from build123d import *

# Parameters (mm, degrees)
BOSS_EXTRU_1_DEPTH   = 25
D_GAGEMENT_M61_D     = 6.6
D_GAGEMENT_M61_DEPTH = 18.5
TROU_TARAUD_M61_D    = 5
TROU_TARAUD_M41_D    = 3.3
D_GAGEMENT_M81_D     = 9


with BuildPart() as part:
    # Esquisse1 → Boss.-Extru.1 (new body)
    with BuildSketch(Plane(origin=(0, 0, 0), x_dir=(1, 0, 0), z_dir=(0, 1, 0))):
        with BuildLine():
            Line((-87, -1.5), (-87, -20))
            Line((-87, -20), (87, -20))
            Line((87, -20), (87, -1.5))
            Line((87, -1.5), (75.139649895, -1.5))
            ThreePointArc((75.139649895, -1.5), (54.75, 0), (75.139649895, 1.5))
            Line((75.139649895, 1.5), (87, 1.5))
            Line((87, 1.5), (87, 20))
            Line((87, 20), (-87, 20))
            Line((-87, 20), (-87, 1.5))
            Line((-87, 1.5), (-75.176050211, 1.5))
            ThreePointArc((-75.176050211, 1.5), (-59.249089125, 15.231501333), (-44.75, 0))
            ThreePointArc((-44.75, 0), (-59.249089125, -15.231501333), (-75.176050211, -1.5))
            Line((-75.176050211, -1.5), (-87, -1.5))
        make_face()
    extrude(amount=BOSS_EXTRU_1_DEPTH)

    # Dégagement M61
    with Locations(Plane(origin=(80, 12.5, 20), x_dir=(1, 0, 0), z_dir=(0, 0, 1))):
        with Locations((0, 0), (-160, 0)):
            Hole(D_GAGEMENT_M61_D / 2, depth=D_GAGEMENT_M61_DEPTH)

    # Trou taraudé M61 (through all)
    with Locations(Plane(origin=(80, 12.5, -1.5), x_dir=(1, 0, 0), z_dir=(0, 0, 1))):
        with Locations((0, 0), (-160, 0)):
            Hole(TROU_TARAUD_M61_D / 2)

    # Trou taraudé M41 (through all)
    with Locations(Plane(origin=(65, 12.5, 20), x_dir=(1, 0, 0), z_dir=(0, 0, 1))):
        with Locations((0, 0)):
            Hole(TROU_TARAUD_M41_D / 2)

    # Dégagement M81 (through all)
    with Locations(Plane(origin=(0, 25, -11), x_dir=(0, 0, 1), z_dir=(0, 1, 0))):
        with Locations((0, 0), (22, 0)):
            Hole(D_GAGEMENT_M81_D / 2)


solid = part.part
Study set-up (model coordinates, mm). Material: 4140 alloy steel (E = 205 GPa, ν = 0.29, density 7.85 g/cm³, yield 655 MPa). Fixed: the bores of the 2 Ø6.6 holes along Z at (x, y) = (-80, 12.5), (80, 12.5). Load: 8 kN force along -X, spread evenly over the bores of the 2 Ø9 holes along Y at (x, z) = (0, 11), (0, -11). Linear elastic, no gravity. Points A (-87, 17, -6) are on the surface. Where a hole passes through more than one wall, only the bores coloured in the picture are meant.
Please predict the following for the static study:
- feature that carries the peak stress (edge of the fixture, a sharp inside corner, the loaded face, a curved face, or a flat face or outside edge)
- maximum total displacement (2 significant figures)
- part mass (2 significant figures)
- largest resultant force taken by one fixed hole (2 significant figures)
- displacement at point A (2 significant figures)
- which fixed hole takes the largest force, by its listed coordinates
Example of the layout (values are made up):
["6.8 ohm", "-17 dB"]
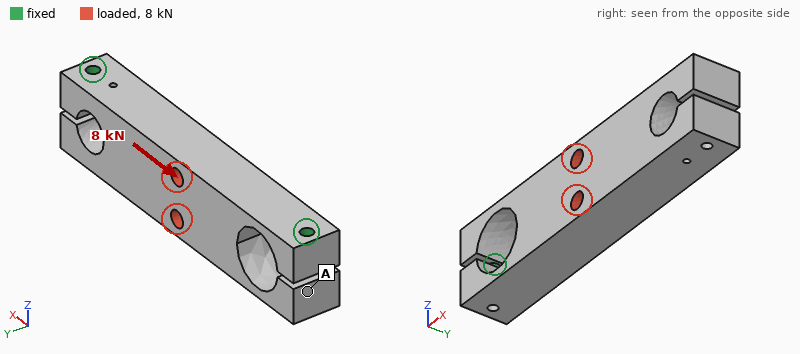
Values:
["a curved face", "20 µm", "1.1 kg", "5.2 kN", "20 µm", "(80, 12.5)"]
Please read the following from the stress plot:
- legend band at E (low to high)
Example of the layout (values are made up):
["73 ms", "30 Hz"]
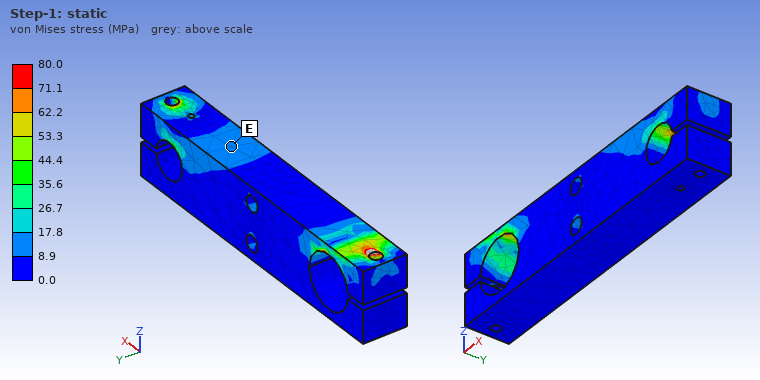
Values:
["8.9 to 17.8 MPa"]
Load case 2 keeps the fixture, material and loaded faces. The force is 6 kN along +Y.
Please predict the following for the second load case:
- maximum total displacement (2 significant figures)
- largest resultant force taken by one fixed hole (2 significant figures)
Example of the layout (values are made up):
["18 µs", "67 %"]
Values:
["0.15 mm", "3.1 kN"]
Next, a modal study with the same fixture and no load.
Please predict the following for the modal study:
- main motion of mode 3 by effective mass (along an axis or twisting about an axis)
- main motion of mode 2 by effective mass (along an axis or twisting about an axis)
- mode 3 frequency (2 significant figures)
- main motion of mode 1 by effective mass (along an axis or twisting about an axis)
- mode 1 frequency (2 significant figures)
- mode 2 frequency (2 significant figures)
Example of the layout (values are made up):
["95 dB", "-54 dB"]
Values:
["along Z", "along Z", "2400 Hz", "along Y", "1200 Hz", "1600 Hz"]
